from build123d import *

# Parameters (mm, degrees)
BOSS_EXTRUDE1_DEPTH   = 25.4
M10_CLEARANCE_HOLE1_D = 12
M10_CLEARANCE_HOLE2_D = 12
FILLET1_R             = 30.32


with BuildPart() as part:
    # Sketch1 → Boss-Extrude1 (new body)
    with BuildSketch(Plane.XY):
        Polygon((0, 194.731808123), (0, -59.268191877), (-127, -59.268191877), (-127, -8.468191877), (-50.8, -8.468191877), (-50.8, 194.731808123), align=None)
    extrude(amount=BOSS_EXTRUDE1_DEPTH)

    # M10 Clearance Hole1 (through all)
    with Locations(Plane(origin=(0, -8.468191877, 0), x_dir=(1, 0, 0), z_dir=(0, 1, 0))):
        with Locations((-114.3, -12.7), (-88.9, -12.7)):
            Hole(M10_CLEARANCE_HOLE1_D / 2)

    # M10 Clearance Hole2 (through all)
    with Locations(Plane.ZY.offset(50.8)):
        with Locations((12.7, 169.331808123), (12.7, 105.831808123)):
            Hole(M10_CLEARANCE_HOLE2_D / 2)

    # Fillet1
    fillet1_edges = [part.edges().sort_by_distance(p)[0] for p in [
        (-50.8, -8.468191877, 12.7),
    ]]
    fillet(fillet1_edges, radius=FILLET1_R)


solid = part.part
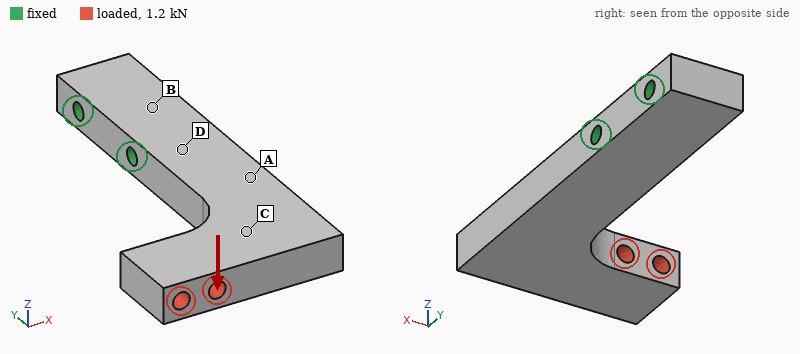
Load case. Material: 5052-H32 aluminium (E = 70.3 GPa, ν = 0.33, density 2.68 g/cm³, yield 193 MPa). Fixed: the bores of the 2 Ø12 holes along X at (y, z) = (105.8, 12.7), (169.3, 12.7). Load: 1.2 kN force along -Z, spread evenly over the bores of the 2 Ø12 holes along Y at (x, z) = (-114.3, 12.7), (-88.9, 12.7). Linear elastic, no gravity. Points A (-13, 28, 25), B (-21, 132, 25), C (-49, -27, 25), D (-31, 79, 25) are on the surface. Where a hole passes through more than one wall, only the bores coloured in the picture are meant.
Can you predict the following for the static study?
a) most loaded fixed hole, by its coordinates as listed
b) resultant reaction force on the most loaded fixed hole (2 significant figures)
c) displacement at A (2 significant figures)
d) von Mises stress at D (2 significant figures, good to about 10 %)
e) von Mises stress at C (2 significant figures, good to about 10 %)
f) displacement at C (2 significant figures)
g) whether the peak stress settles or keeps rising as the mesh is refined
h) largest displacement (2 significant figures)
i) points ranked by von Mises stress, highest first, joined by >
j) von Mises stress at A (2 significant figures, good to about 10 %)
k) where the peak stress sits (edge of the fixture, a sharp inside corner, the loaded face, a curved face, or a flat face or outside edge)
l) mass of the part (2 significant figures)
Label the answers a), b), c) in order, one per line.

a) (105.8, 12.7)
b) 1.8 kN
c) 0.081 mm
d) 30 MPa
e) 9.2 MPa
f) 0.27 mm
g) keeps rising
h) 0.53 mm
i) D > A > C > B
j) 20 MPa
k) edge of the fixture
l) 1.1 kg
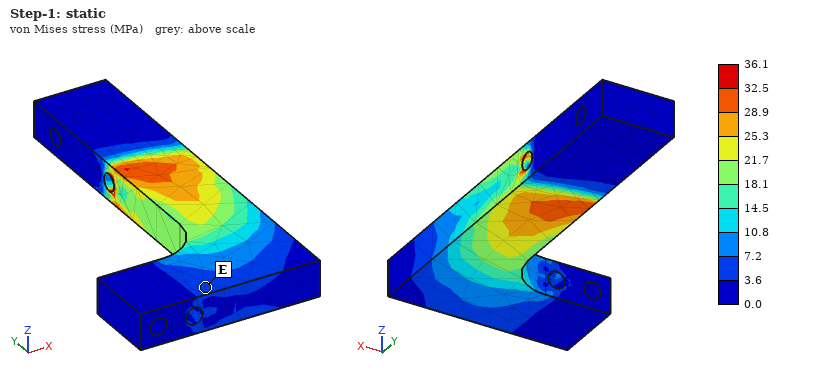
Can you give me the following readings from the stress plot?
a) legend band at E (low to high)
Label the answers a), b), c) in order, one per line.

a) 3.6 to 7.2 MPa
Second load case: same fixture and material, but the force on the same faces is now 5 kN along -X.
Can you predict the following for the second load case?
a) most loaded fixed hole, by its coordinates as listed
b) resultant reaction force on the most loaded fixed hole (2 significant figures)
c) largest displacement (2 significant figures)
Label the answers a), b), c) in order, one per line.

a) (105.8, 12.7)
b) 5.4 kN
c) 0.39 mm
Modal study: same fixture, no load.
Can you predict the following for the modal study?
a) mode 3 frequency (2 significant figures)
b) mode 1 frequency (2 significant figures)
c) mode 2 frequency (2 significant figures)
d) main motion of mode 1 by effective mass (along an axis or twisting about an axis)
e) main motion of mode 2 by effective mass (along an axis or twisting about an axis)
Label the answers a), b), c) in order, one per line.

a) 1300 Hz
b) 490 Hz
c) 950 Hz
d) along Z
e) along X
